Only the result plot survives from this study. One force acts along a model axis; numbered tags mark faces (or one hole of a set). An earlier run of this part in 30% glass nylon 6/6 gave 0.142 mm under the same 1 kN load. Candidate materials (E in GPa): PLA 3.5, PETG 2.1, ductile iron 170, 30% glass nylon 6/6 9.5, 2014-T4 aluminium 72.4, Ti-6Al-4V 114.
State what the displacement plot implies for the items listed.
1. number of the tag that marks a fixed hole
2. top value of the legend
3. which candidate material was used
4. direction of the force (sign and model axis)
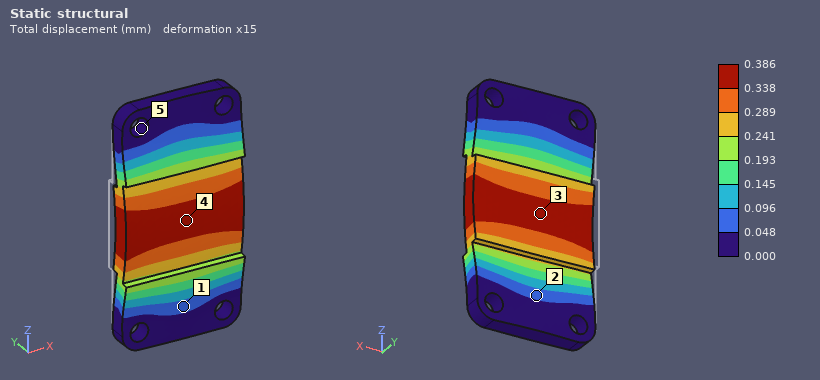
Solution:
5
0.386 mm
PLA
-Y
